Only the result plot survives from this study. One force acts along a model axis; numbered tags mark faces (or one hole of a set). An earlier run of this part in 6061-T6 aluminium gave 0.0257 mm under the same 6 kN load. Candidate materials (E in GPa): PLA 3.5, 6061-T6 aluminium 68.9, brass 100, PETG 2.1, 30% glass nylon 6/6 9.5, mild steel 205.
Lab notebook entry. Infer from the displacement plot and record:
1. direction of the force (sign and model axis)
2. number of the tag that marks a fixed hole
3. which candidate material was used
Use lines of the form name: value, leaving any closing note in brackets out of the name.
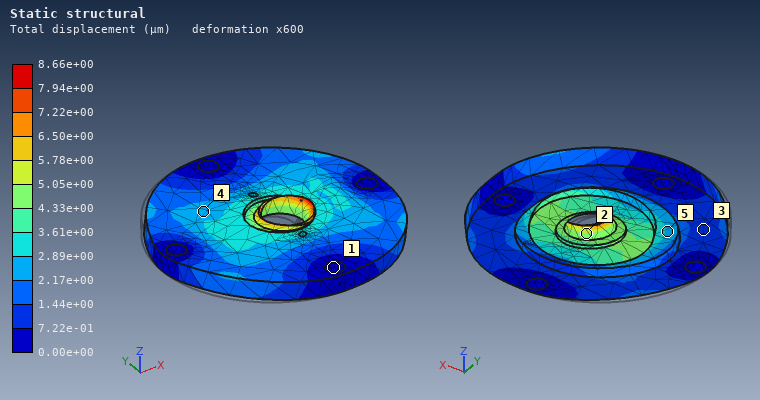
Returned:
direction of the force: +X
number of the tag that marks a fixed hole: 1
which candidate material was used: mild steel
